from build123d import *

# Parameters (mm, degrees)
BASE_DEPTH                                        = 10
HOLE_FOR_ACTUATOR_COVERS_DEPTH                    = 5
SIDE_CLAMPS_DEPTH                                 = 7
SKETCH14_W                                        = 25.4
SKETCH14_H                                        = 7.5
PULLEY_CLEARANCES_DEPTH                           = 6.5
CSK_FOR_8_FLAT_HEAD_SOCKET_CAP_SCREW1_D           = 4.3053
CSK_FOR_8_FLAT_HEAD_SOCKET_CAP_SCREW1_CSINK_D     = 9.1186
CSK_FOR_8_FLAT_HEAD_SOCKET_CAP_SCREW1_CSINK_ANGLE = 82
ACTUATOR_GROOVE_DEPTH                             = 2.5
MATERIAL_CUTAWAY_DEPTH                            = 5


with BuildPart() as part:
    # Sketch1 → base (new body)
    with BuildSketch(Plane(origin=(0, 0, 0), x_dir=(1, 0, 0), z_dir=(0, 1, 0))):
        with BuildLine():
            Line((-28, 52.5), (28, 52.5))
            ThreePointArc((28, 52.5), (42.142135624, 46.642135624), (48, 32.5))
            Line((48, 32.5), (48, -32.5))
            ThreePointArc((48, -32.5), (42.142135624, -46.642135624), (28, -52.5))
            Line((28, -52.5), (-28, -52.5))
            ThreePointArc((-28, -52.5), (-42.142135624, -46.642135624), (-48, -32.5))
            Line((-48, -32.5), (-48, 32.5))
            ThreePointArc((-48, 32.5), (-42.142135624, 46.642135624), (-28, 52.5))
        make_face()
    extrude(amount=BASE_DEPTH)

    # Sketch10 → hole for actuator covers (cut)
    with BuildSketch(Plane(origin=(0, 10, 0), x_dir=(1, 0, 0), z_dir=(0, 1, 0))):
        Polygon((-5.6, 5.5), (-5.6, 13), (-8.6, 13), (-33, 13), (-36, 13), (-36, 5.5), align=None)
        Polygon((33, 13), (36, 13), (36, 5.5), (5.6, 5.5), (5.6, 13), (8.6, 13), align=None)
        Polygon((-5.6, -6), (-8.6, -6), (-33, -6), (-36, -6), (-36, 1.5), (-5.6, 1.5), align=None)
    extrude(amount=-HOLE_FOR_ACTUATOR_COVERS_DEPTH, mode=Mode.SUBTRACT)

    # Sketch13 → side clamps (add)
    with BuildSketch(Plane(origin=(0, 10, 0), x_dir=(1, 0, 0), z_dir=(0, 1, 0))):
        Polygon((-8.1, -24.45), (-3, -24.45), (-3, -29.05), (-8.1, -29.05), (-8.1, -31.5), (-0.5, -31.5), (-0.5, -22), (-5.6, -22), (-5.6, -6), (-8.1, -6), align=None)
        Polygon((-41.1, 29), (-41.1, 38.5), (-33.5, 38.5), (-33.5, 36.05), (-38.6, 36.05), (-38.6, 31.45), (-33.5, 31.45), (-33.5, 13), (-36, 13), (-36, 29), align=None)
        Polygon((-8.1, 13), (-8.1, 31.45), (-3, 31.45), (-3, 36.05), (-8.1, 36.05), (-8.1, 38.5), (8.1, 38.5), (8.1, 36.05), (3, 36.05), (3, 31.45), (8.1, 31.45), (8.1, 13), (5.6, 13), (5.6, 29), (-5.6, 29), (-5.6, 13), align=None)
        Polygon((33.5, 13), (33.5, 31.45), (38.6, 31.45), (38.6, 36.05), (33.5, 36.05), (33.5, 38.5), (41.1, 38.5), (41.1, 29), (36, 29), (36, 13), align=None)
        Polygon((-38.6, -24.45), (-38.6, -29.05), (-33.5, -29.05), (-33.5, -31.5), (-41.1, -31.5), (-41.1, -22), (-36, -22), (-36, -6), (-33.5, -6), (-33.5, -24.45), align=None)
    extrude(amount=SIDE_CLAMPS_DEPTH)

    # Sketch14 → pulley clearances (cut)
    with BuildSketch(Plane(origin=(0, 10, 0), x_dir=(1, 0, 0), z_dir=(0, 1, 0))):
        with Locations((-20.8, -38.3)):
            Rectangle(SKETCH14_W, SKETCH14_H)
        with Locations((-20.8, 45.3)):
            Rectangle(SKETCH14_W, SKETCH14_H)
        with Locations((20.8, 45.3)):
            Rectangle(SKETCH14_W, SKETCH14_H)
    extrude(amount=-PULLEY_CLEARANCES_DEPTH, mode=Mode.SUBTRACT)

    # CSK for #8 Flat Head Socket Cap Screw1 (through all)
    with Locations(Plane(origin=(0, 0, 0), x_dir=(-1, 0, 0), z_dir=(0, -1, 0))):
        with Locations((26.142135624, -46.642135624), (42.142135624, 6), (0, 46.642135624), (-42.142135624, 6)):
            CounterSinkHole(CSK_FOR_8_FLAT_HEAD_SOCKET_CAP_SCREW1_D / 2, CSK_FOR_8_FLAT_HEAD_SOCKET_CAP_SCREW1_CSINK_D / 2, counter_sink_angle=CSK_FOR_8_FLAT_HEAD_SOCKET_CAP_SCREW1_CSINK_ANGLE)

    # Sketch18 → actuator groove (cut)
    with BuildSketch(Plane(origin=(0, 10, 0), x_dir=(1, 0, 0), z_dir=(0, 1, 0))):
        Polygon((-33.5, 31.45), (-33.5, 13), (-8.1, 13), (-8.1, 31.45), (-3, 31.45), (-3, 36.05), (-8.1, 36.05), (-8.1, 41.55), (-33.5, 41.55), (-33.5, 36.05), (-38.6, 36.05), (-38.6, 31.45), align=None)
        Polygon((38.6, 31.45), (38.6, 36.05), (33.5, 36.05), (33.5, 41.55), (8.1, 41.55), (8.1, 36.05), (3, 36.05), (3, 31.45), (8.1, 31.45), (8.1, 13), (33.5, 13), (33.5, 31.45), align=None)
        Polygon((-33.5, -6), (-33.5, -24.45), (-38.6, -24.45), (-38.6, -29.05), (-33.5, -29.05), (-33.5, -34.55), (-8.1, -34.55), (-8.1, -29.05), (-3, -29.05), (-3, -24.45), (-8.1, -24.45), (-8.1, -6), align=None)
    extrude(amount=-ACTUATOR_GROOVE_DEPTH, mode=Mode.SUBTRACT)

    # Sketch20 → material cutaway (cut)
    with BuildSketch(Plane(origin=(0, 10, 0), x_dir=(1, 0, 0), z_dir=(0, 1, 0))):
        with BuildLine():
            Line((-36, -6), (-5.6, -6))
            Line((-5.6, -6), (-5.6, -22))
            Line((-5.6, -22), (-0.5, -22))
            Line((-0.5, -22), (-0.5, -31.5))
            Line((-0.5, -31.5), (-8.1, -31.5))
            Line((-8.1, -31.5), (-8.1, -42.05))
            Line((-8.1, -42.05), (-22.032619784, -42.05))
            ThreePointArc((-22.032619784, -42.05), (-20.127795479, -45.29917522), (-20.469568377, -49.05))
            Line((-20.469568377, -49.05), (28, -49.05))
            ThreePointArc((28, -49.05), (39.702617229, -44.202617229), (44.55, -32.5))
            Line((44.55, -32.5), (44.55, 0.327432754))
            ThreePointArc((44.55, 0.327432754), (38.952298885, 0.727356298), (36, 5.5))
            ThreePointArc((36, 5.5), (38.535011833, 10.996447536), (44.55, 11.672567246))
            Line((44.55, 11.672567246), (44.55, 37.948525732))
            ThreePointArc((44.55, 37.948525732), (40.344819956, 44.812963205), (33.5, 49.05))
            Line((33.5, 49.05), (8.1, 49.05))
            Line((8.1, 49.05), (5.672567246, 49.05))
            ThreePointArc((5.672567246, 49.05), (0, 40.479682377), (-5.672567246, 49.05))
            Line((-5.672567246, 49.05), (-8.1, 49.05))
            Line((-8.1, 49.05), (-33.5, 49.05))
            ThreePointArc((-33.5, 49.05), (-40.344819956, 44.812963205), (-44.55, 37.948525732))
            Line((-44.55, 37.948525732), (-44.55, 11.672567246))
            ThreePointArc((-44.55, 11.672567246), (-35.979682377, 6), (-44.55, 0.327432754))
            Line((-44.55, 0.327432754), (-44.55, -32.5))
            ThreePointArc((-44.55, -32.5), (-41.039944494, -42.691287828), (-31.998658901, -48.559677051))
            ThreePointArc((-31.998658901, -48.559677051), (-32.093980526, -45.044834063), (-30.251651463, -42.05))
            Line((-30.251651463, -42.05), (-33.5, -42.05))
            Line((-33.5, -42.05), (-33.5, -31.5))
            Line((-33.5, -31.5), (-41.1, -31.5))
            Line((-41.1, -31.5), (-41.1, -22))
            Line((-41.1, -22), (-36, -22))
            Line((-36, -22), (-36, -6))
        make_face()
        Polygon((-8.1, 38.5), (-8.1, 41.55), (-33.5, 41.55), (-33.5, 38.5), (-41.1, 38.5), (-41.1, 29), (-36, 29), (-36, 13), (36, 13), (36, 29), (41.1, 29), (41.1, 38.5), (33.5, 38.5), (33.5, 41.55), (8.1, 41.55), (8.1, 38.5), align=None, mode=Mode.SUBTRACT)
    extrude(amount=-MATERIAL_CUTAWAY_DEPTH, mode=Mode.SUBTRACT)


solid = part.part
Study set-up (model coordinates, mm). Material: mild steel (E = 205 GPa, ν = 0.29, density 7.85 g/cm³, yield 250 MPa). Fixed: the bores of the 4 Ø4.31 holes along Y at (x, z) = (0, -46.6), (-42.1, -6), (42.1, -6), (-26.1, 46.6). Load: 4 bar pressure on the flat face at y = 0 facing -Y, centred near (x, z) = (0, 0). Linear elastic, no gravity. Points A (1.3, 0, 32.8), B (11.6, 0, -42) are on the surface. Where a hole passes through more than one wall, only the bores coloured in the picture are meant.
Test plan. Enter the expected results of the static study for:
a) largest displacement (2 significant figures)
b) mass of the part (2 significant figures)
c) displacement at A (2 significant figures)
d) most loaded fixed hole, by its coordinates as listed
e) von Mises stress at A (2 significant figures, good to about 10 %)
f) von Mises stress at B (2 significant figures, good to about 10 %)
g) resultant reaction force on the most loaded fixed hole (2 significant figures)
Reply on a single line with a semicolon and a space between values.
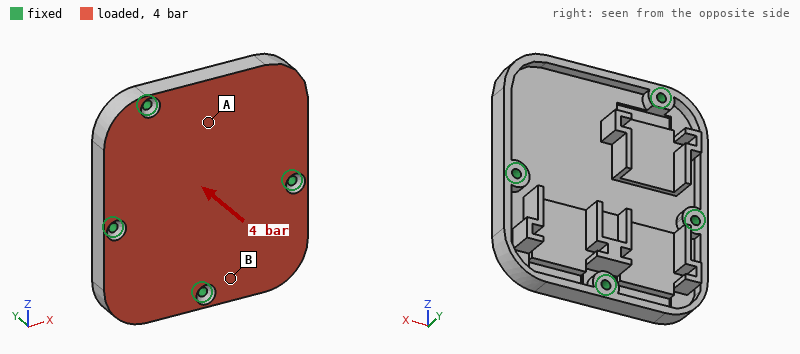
54 µm; 530 g; 23 µm; (42.1, -6); 19 MPa; 9.4 MPa; 1.5 kN
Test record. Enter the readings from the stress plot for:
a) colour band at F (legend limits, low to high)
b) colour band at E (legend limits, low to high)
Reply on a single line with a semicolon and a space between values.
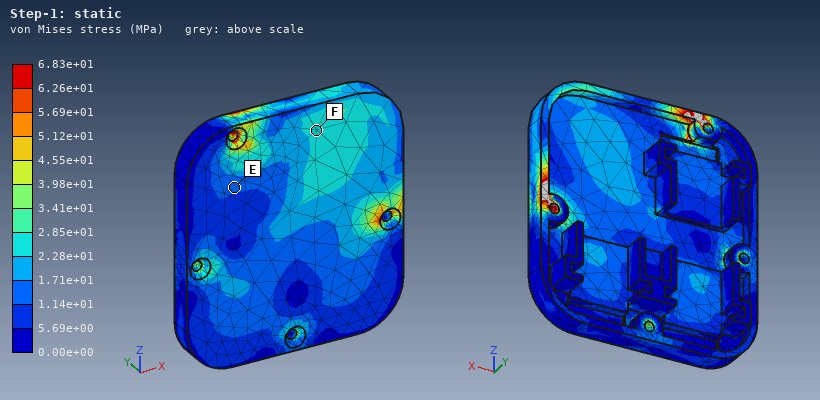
2.28e+01 to 2.85e+01 MPa; 1.14e+01 to 1.71e+01 MPa
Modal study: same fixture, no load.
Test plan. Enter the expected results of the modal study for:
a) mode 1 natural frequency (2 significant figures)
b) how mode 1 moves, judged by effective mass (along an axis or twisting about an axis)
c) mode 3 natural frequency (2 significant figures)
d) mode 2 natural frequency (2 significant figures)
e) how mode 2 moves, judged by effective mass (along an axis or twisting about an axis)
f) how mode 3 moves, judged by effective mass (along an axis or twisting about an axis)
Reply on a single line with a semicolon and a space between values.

2600 Hz; along Y; 5300 Hz; 4500 Hz; along Y; twisting about Z
